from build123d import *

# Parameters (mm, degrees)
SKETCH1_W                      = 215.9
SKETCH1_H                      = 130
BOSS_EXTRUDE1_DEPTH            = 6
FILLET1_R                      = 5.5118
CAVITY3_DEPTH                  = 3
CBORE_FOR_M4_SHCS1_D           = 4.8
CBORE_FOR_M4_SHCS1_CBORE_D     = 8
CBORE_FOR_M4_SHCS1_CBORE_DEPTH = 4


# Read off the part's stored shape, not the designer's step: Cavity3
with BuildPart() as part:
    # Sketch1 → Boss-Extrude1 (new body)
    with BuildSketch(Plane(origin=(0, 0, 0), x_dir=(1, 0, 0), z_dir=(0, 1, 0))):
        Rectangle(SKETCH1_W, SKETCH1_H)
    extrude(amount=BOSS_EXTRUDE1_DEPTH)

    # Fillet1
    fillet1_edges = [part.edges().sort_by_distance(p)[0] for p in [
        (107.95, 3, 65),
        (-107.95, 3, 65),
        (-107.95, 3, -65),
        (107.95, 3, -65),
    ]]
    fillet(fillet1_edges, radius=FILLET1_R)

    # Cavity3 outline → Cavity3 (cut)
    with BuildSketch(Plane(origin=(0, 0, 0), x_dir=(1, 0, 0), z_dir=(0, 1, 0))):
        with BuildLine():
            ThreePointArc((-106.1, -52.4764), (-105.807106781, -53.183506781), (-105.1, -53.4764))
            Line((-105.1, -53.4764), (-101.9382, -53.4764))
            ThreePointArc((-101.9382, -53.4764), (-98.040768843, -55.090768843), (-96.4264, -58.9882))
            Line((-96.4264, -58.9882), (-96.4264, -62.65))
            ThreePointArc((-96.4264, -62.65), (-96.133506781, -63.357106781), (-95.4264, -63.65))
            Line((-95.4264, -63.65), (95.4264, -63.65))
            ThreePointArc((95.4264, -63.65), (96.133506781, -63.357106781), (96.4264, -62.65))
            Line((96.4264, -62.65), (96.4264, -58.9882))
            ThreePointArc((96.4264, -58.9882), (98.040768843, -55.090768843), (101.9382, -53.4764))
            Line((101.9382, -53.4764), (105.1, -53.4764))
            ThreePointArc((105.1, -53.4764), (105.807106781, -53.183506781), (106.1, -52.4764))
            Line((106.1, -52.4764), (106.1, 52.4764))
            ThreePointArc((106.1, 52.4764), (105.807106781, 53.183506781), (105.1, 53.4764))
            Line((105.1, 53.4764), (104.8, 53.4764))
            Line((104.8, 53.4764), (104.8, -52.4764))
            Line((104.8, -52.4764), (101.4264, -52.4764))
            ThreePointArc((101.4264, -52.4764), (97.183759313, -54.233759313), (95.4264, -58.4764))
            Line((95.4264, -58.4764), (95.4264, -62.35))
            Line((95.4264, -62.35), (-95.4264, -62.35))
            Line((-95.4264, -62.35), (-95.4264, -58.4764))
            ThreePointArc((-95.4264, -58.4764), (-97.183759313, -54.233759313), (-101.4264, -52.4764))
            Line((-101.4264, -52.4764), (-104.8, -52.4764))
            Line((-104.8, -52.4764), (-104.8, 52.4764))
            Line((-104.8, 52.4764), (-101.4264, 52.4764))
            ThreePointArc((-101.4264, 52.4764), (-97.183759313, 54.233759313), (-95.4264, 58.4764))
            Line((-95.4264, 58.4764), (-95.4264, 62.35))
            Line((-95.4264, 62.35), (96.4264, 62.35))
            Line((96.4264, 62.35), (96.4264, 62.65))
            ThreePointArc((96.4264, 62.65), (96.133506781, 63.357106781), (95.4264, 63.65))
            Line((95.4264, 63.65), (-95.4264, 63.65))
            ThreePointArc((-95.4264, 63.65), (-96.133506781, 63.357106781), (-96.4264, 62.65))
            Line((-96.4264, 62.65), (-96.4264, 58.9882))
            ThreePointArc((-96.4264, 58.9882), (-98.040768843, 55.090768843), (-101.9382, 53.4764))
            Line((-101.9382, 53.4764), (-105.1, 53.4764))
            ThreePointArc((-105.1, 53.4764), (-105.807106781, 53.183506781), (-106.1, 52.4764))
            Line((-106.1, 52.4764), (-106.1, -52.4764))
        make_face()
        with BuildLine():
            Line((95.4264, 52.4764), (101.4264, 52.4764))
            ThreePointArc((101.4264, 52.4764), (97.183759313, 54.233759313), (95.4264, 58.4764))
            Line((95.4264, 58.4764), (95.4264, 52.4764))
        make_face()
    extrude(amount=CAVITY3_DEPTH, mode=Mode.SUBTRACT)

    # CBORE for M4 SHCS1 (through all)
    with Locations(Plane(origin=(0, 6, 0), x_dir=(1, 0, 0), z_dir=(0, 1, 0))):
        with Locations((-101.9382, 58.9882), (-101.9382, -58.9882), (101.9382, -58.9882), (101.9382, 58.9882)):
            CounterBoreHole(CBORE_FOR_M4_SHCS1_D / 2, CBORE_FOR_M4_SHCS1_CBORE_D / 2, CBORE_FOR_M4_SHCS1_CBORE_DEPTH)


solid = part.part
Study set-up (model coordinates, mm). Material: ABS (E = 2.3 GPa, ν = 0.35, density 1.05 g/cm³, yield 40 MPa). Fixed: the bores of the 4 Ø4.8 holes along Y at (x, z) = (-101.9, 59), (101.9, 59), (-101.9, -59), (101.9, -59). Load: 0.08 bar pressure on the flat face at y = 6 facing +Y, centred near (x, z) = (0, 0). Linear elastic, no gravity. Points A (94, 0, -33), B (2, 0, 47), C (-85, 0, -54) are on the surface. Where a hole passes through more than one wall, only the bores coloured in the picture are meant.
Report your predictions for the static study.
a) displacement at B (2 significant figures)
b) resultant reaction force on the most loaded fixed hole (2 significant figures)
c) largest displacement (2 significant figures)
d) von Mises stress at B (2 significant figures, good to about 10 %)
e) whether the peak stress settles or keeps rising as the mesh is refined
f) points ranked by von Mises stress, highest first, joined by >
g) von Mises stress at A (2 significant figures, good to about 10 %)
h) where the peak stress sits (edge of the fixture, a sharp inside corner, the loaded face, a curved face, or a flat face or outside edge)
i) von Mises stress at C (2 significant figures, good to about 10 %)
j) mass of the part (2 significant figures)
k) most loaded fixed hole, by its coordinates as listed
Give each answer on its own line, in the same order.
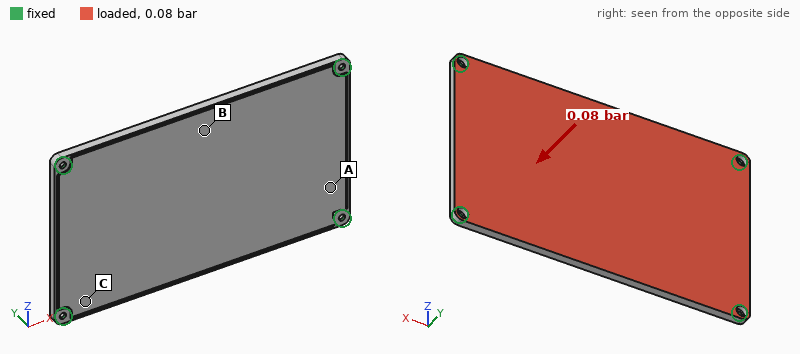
2.5 mm
130 N
2.6 mm
4.3 MPa
keeps rising
B > C > A
1.3 MPa
edge of the fixture
2.5 MPa
170 g
(101.9, -59)
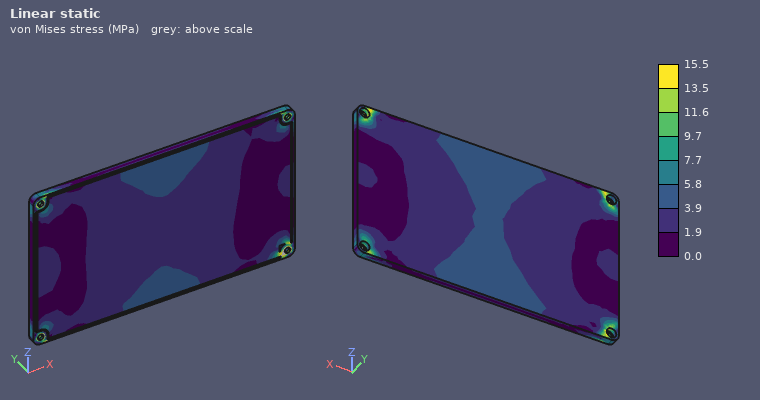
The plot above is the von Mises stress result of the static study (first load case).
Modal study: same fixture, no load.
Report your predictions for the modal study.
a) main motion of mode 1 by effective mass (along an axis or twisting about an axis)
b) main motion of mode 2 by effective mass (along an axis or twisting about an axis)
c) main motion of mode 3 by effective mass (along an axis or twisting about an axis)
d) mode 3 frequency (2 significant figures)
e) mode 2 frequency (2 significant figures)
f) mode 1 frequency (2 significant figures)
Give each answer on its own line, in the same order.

along Y
twisting about X
twisting about Z
370 Hz
260 Hz
130 Hz
